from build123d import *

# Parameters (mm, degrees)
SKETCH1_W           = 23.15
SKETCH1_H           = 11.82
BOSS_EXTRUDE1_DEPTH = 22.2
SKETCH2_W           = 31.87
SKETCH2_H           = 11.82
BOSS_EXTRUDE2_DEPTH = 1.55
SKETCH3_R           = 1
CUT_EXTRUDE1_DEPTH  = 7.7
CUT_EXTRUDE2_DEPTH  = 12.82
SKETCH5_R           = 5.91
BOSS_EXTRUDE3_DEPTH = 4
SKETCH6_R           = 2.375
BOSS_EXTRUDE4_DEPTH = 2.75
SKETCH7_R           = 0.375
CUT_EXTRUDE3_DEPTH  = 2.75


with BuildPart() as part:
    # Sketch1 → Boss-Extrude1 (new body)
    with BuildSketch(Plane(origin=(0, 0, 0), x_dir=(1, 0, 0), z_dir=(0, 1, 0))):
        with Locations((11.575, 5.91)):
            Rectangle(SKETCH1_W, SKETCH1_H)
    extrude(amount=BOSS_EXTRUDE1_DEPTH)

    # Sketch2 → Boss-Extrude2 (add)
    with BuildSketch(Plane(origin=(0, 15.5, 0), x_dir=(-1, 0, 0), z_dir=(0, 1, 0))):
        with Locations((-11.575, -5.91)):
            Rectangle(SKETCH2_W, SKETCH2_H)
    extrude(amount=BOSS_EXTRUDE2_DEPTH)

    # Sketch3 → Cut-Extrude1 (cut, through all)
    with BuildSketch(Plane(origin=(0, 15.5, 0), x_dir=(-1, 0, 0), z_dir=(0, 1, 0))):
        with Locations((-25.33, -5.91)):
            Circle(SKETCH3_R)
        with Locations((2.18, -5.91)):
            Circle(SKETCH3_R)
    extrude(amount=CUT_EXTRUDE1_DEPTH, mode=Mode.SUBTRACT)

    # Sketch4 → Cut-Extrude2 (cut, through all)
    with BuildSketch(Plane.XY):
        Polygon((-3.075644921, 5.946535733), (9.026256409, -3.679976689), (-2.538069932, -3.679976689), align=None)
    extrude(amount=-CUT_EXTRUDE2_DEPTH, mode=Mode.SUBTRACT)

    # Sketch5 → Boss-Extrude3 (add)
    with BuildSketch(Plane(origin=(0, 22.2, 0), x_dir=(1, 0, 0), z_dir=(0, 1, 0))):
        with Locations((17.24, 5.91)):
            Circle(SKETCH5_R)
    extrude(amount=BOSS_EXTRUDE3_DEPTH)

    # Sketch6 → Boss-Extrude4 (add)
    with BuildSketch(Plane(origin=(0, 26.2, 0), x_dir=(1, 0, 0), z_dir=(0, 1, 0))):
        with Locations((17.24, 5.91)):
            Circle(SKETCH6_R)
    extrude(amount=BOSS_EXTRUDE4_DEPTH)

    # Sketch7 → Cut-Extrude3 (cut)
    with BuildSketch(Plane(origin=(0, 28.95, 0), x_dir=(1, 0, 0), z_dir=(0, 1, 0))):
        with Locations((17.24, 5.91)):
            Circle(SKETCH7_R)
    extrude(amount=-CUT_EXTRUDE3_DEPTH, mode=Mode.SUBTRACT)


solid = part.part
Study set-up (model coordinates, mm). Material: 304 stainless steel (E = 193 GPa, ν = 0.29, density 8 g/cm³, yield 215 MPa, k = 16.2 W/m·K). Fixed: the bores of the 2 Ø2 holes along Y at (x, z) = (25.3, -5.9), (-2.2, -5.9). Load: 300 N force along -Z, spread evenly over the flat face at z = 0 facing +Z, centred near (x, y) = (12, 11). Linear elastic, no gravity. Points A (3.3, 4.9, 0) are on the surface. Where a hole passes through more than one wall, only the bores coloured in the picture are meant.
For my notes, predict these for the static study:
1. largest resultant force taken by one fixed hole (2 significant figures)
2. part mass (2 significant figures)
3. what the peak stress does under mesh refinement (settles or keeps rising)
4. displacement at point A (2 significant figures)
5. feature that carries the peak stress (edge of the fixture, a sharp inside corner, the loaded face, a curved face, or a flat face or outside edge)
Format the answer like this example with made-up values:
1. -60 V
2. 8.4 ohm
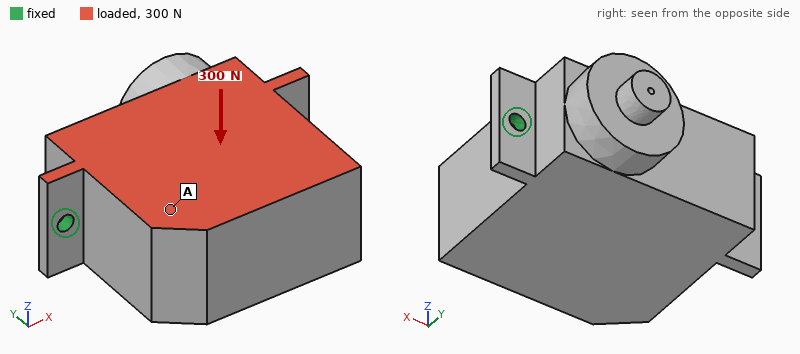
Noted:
1. 150 N
2. 53 g
3. keeps rising
4. 19 µm
5. edge of the fixture
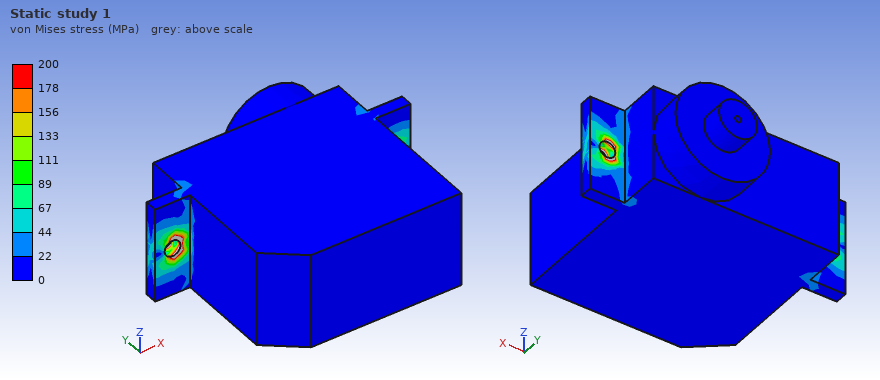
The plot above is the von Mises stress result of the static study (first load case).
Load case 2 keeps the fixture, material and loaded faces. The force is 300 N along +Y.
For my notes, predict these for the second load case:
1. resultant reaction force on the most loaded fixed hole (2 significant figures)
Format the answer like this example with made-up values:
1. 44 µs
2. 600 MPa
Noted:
1. 150 N
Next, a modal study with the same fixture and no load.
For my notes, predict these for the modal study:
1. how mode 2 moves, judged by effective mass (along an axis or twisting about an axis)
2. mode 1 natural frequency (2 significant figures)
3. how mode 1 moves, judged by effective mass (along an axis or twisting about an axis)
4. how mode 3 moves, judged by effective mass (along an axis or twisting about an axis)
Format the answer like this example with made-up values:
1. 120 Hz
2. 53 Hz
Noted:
1. along Y
2. 2600 Hz
3. along Z
4. along X
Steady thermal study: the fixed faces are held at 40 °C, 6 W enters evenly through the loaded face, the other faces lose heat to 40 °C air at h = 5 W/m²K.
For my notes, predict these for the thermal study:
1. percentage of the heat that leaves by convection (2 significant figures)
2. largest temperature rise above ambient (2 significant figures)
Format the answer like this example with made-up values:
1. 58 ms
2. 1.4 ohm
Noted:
1. 6.6 %
2. 51 K
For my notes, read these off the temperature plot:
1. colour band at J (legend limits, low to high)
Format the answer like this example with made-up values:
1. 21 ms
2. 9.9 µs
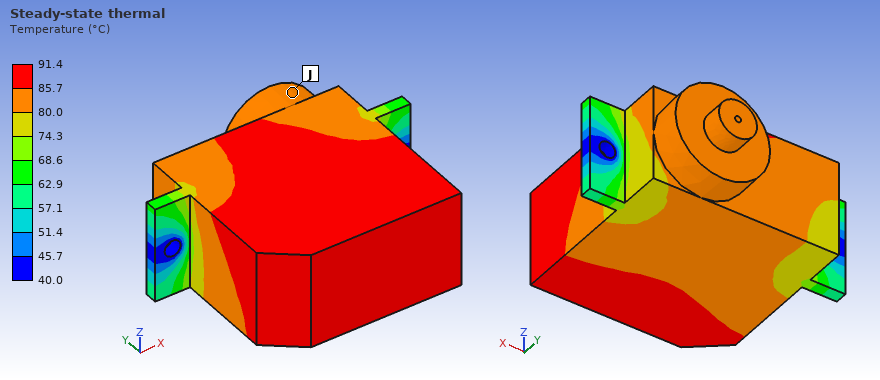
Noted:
1. 80.0 to 85.7 °C
